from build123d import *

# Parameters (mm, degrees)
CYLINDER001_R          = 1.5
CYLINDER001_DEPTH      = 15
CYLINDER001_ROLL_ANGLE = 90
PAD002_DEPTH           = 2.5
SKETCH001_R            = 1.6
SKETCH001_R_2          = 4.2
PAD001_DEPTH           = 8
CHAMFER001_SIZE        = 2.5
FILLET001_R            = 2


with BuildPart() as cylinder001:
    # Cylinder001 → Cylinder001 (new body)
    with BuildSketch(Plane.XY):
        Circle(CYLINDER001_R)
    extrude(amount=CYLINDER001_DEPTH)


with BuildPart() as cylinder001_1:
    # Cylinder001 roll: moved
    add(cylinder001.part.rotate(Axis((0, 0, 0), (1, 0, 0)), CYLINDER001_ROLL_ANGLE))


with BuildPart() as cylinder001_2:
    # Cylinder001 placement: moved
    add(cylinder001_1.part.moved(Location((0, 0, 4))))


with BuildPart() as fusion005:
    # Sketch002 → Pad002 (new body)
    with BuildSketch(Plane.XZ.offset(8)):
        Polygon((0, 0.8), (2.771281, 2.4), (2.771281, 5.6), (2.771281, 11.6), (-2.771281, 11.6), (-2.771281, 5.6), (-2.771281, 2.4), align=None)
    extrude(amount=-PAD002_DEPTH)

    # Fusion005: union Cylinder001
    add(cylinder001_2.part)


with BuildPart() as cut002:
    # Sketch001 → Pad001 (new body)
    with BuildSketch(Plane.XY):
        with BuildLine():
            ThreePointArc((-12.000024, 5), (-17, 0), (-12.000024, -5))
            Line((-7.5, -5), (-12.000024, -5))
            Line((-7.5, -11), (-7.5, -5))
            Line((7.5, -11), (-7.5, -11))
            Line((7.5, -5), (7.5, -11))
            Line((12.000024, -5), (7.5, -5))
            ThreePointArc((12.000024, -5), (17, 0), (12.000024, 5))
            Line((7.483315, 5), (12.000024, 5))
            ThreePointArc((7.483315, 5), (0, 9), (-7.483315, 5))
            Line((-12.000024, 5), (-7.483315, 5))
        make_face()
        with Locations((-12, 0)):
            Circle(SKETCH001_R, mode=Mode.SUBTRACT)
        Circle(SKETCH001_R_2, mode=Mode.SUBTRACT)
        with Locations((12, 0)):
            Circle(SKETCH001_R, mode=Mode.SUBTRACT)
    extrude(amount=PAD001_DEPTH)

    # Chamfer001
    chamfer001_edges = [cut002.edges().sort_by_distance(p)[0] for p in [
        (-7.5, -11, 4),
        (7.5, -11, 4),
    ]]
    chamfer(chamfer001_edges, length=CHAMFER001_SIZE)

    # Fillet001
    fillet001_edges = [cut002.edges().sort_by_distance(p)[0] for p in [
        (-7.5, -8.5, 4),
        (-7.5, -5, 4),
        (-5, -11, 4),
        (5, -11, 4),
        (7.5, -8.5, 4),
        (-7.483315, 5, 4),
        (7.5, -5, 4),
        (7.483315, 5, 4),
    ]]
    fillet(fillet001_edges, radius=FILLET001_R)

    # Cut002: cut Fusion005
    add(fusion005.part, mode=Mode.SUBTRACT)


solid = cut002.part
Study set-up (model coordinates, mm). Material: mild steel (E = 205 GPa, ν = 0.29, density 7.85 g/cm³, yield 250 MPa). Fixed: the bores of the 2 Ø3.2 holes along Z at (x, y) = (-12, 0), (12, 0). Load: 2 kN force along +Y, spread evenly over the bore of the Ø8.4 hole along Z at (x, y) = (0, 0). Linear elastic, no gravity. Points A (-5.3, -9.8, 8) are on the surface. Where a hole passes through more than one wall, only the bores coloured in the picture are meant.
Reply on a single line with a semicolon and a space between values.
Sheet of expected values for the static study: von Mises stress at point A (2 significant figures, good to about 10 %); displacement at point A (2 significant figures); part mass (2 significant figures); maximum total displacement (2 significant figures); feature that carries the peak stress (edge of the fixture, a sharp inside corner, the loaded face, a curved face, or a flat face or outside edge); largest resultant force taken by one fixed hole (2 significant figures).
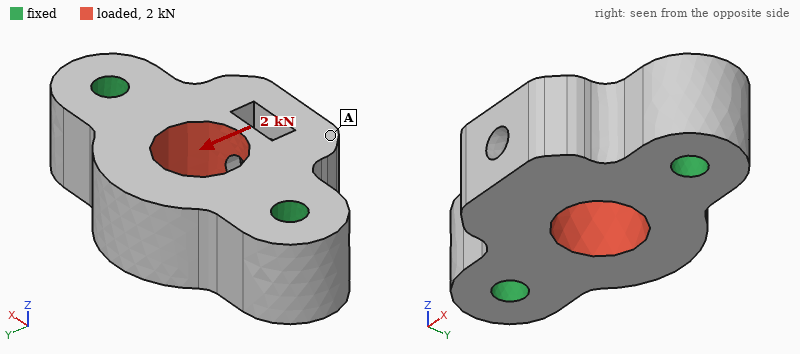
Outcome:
11 MPa; 1.3 µm; 23 g; 2.4 µm; a curved face; 1.0 kN
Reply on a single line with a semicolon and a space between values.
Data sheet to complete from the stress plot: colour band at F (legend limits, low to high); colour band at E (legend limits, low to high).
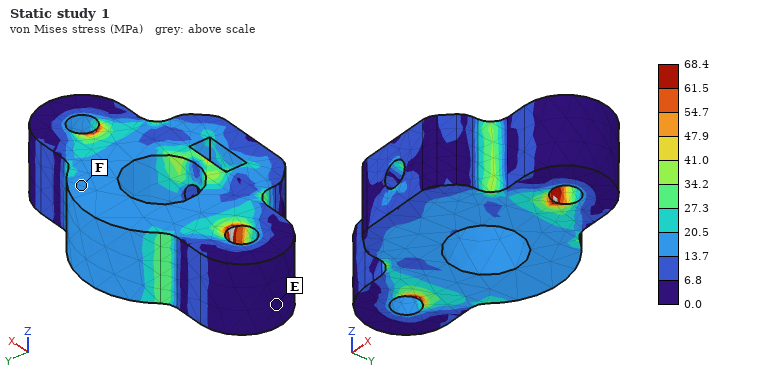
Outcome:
13.7 to 20.5 MPa; 0.0 to 6.8 MPa
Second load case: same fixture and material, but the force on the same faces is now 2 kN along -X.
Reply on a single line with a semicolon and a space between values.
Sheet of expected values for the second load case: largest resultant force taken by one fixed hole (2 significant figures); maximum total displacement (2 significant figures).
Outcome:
1.0 kN; 0.80 µm
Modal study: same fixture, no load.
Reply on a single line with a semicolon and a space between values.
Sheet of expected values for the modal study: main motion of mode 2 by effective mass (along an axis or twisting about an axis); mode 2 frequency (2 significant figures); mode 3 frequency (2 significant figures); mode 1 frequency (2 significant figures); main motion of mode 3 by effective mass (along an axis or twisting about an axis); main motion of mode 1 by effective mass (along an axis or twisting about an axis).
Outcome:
along Z; 40 kHz; 52 kHz; 31 kHz; along Y; along Z
